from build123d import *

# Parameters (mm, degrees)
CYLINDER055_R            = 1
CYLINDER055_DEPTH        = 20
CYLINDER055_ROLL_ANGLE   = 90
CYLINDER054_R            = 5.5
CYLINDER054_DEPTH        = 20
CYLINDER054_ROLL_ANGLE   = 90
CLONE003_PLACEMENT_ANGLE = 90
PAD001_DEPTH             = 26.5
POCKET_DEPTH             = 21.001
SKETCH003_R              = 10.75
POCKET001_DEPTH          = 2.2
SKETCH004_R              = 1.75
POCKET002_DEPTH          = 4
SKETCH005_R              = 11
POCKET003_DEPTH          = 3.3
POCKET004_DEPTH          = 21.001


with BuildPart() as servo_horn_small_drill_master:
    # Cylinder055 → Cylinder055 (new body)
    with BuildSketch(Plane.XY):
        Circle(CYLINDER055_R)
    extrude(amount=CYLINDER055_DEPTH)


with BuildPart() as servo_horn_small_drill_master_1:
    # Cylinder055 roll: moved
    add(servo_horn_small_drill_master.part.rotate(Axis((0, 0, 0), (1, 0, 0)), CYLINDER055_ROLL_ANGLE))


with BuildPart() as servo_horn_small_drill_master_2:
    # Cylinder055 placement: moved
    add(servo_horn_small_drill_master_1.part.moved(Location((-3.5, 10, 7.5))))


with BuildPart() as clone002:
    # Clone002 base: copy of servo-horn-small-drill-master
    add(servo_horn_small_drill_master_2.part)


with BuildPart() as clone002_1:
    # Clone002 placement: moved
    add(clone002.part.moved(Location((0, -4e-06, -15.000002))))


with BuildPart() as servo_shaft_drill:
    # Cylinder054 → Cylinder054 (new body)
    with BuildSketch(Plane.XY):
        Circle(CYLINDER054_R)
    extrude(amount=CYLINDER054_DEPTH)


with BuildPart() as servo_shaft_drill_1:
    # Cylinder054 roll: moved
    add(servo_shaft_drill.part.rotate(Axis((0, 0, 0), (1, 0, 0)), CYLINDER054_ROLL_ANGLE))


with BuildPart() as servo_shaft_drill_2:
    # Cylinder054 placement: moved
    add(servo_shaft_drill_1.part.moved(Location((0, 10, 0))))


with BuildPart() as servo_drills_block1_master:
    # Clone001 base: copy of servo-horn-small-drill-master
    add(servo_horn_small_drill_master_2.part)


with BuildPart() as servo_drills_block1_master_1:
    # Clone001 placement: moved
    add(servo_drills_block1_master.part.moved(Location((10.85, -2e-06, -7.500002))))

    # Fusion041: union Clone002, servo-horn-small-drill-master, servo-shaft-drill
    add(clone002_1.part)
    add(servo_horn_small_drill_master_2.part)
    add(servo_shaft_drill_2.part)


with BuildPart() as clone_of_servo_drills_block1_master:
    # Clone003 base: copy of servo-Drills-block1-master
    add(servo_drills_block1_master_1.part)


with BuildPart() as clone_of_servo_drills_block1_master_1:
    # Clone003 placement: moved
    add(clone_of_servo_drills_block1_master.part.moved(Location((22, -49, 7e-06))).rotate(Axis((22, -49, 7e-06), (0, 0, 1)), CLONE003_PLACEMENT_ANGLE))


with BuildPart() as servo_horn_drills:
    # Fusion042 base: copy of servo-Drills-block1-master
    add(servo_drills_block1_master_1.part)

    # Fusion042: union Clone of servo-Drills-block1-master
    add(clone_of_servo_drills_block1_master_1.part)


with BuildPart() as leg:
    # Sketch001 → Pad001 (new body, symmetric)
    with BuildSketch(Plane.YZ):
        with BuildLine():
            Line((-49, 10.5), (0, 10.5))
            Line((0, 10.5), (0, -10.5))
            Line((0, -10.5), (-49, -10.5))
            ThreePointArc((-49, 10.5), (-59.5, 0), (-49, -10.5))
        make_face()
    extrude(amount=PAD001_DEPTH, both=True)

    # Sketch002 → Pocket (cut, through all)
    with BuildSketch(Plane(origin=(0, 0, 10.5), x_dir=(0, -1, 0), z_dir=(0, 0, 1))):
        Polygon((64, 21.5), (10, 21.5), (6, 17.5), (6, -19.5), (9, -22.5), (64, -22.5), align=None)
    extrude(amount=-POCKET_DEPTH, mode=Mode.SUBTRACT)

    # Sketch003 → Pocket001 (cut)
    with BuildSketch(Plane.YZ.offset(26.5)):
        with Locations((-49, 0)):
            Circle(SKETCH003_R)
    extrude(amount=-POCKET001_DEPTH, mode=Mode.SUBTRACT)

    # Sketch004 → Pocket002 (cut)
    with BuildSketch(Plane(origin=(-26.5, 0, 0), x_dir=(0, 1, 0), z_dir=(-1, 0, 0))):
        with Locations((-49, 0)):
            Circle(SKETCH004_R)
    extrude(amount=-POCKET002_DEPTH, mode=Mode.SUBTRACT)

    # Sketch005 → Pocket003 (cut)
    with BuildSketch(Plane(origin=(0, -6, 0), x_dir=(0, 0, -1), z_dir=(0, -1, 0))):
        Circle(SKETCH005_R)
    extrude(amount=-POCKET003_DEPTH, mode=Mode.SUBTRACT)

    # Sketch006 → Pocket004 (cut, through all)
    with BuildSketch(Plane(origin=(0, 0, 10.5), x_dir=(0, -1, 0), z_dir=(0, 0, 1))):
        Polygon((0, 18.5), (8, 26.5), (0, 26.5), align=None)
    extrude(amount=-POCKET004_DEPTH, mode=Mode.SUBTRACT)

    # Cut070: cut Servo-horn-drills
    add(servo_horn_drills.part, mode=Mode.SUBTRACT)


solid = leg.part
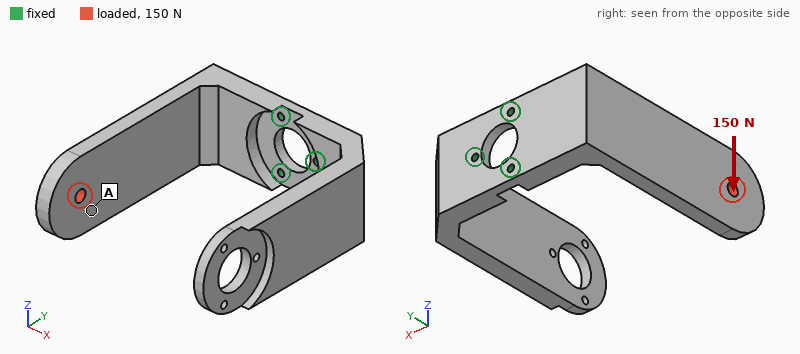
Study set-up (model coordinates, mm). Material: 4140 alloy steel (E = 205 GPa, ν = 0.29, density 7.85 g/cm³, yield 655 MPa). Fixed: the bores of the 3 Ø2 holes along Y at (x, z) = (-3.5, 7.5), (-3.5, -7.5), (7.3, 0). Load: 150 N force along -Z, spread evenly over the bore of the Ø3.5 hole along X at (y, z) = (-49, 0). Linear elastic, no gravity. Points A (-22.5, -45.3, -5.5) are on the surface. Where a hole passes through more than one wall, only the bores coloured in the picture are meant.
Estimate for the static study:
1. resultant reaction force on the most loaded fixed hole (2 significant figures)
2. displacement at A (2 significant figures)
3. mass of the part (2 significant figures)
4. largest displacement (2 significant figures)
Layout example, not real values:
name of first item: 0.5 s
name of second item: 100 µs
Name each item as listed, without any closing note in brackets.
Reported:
resultant reaction force on the most loaded fixed hole: 450 N
displacement at A: 0.083 mm
mass of the part: 100 g
largest displacement: 0.11 mm
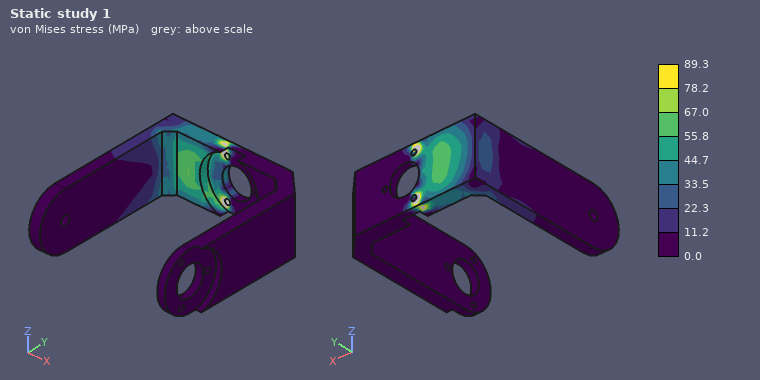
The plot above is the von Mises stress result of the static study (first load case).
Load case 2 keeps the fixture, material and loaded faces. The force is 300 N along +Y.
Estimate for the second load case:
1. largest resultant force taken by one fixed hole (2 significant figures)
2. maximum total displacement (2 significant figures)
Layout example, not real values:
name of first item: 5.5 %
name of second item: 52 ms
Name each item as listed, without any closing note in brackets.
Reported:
largest resultant force taken by one fixed hole: 170 N
maximum total displacement: 0.31 mm
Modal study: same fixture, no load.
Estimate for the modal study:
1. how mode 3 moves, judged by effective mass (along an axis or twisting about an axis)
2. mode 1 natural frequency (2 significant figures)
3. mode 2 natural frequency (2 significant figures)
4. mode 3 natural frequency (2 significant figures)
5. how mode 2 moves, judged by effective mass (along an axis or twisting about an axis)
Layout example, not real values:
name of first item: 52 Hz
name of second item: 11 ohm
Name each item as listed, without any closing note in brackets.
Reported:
how mode 3 moves, judged by effective mass: along Z
mode 1 natural frequency: 650 Hz
mode 2 natural frequency: 980 Hz
mode 3 natural frequency: 1300 Hz
how mode 2 moves, judged by effective mass: along X
